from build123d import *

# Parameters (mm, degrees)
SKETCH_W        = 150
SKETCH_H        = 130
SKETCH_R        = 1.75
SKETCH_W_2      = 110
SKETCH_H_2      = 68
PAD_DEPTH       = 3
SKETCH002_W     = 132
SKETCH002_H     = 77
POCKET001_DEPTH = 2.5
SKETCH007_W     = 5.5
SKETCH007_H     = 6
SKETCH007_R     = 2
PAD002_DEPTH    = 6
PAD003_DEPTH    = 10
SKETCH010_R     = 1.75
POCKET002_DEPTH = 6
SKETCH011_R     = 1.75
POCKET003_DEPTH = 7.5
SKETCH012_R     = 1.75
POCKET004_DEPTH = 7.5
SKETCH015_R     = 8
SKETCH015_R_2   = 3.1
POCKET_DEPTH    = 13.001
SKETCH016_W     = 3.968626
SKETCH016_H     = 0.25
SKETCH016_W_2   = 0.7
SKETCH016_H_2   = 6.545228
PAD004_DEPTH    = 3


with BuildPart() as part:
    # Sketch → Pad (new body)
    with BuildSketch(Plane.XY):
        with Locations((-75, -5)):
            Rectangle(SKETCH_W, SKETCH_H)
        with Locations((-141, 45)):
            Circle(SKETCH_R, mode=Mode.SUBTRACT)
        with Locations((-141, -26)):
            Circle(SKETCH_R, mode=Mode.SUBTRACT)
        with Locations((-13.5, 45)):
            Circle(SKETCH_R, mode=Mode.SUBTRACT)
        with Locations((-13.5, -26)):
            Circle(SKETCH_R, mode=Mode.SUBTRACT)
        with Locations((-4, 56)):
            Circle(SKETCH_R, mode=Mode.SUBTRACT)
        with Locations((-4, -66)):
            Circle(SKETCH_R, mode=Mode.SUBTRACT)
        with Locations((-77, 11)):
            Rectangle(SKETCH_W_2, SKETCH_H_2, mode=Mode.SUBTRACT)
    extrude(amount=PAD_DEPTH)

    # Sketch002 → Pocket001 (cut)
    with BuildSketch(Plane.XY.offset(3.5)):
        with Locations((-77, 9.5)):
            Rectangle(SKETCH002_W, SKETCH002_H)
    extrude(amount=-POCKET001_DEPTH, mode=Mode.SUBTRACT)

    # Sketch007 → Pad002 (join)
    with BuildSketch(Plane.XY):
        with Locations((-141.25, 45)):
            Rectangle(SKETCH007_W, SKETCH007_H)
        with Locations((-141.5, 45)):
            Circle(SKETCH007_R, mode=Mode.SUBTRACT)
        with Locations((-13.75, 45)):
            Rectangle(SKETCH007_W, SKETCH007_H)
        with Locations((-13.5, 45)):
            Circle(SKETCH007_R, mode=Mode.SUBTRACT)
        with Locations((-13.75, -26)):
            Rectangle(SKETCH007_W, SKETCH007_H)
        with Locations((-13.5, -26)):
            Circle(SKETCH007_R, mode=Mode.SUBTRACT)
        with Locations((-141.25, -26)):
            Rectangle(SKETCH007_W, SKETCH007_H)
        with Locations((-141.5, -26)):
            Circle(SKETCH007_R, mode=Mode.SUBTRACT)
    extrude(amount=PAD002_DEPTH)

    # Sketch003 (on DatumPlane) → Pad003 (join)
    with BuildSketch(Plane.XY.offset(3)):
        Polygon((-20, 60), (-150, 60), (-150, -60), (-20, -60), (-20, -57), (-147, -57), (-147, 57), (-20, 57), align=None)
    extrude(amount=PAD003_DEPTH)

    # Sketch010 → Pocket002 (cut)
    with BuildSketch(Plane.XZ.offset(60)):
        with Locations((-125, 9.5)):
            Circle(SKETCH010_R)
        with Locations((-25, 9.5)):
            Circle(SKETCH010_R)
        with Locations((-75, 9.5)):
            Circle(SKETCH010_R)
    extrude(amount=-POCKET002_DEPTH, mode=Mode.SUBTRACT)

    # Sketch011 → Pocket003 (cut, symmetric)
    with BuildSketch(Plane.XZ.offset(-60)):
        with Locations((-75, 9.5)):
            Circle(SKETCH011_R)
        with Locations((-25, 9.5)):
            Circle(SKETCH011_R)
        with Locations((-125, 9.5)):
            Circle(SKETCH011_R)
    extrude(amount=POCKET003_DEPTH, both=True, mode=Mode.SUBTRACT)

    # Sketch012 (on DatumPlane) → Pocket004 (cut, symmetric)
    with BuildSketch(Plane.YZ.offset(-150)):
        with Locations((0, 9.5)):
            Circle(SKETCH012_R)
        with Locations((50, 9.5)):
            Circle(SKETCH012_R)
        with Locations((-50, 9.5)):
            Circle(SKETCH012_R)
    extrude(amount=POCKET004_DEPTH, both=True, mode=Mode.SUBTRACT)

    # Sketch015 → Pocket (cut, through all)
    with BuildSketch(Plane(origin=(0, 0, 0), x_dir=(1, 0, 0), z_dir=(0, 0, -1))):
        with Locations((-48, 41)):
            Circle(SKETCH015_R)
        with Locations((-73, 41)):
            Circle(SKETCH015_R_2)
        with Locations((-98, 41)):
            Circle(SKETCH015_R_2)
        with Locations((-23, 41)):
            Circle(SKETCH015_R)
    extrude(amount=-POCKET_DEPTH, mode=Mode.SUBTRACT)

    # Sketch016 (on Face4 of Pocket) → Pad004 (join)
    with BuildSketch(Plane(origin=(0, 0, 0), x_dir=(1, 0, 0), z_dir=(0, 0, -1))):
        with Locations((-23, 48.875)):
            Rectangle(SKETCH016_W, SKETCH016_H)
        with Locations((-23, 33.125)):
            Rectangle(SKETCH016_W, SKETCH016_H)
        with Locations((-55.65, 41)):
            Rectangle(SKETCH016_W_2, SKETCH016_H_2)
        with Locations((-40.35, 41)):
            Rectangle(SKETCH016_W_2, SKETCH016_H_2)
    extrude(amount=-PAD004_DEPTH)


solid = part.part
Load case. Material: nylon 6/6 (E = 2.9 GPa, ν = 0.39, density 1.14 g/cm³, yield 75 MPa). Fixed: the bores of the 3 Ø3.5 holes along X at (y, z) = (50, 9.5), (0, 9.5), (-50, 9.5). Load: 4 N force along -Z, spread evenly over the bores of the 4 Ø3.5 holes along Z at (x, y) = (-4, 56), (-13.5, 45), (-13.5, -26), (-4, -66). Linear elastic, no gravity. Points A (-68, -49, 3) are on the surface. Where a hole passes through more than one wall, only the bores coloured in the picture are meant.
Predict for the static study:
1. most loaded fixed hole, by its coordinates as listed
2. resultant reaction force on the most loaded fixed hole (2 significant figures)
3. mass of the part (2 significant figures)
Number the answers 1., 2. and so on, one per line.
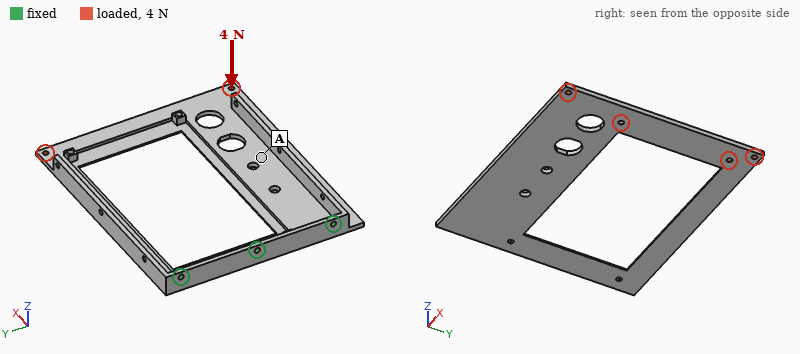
1. (0, 9.5)
2. 11 N
3. 46 g
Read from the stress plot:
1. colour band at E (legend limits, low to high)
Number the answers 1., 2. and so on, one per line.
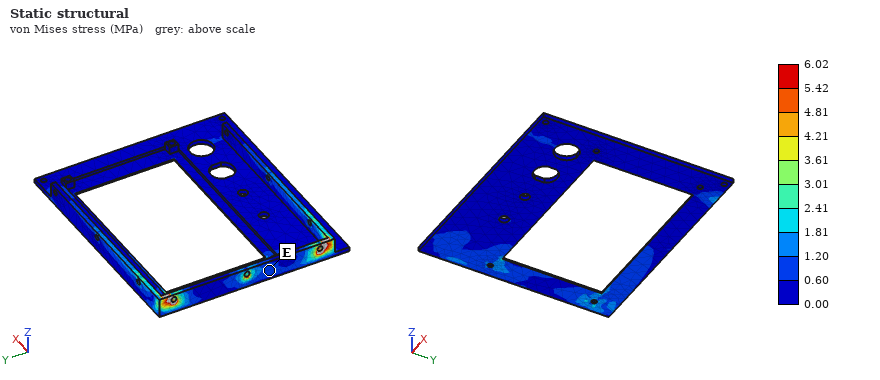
1. 0.60 to 1.20 MPa
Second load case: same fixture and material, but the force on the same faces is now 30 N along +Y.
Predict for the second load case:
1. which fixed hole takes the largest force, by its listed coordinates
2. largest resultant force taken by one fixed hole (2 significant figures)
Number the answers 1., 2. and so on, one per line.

1. (-50, 9.5)
2. 53 N
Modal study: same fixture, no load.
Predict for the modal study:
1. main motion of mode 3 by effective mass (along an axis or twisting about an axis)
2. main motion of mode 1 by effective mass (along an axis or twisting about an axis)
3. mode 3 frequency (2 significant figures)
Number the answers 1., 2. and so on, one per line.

1. along Y
2. along Z
3. 240 Hz
